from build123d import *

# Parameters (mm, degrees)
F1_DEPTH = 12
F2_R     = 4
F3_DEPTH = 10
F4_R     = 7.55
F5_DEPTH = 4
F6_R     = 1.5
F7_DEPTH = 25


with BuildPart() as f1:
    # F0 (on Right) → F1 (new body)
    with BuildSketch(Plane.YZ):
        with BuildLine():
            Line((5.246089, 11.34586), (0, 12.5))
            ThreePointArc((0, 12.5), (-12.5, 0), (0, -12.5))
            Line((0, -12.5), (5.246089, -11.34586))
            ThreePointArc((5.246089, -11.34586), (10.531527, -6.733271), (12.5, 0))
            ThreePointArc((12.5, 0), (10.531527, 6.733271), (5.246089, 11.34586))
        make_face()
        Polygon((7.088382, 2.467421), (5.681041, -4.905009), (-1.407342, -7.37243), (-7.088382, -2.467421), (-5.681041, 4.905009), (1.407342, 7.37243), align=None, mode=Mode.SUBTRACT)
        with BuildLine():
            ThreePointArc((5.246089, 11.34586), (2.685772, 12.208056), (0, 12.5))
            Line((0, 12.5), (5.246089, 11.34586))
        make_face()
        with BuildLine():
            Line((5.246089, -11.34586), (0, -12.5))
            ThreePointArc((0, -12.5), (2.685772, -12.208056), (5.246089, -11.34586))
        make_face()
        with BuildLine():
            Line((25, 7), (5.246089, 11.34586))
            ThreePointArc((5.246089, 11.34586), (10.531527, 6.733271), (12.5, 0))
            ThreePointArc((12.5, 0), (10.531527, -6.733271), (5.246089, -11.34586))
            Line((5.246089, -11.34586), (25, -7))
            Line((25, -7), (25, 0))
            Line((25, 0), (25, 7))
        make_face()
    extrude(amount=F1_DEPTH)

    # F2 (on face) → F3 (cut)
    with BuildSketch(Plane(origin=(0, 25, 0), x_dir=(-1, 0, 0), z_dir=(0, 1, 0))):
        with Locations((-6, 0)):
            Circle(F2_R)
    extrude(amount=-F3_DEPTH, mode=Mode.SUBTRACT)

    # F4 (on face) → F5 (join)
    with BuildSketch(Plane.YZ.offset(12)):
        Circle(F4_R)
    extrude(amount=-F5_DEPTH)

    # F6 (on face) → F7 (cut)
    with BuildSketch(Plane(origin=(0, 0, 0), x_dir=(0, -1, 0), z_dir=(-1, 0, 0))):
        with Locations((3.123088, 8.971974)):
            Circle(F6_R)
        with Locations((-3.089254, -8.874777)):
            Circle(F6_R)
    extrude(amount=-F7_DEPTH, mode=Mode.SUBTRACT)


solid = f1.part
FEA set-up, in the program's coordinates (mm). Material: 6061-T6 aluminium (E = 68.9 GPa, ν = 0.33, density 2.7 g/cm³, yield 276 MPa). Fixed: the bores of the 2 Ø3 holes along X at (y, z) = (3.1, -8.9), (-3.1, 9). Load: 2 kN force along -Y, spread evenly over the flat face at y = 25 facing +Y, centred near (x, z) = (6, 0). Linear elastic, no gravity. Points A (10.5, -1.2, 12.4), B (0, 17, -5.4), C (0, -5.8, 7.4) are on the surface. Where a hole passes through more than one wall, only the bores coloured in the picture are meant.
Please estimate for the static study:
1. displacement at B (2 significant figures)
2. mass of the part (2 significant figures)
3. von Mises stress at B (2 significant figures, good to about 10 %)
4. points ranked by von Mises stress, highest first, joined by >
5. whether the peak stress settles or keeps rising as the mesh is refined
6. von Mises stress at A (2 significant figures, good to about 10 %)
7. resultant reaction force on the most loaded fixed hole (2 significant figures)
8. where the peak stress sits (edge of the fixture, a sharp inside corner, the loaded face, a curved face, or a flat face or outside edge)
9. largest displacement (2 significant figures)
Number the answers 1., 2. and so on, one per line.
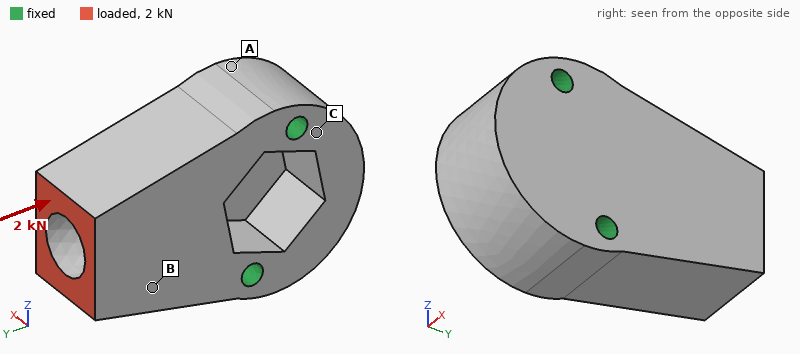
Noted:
1. 3.5 µm
2. 19 g
3. 13 MPa
4. B > A > C
5. keeps rising
6. 5.8 MPa
7. 1.0 kN
8. edge of the fixture
9. 6.6 µm
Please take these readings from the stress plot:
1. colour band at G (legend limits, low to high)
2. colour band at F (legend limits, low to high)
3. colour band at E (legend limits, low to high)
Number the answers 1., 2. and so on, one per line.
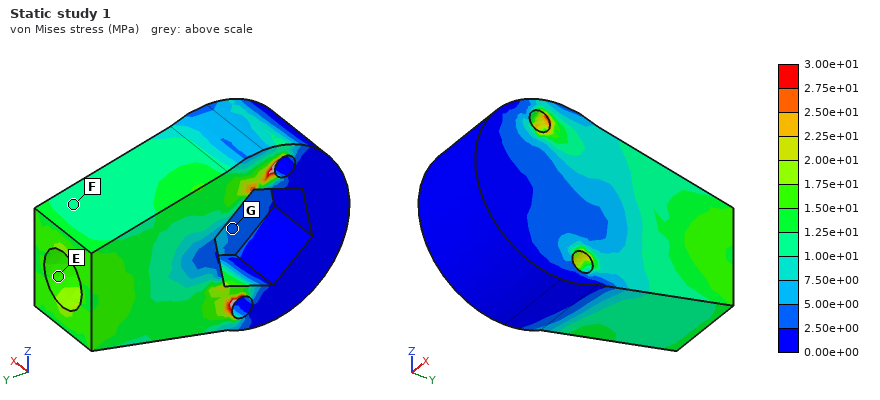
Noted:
1. 2.50e+00 to 5.00e+00 MPa
2. 1.00e+01 to 1.25e+01 MPa
3. 1.50e+01 to 1.75e+01 MPa
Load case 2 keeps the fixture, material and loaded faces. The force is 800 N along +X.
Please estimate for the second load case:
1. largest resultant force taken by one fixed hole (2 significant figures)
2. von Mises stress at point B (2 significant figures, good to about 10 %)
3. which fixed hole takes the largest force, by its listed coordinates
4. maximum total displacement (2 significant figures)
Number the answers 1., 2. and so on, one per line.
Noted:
1. 640 N
2. 21 MPa
3. (3.1, -8.9)
4. 35 µm
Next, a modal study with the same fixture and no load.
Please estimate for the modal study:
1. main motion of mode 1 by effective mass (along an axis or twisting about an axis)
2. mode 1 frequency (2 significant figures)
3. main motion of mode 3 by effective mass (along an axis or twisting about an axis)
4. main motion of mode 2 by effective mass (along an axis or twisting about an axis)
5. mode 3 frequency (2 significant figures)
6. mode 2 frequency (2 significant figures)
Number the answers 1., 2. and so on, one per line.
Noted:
1. along X
2. 15 kHz
3. twisting about Y
4. along Z
5. 32 kHz
6. 25 kHz
